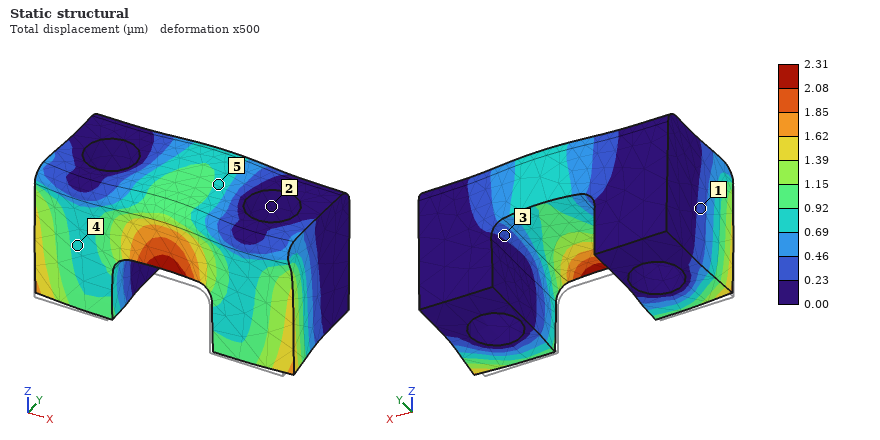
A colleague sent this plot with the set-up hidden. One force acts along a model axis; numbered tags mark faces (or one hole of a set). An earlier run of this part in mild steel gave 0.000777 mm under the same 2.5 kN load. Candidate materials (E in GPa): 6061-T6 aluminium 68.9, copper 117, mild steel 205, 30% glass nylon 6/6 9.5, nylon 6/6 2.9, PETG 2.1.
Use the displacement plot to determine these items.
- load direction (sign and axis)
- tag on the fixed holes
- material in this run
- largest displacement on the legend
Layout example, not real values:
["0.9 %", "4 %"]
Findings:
["+Y", "2", "6061-T6 aluminium", "2.31 µm"]
